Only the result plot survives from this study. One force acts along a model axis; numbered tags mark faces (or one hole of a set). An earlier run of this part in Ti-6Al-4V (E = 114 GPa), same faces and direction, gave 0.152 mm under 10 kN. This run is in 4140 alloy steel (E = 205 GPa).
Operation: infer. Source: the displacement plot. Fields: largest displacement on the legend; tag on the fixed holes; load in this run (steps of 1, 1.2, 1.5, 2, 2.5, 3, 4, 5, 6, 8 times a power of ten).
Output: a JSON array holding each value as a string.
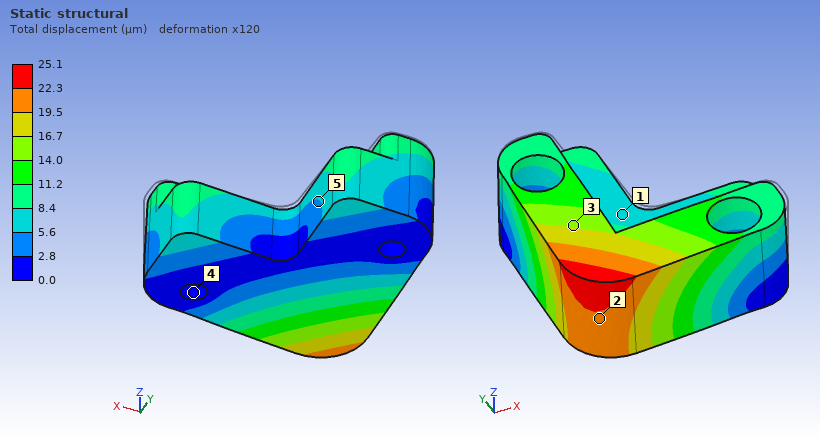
["25.1 µm", "4", "3 kN"]
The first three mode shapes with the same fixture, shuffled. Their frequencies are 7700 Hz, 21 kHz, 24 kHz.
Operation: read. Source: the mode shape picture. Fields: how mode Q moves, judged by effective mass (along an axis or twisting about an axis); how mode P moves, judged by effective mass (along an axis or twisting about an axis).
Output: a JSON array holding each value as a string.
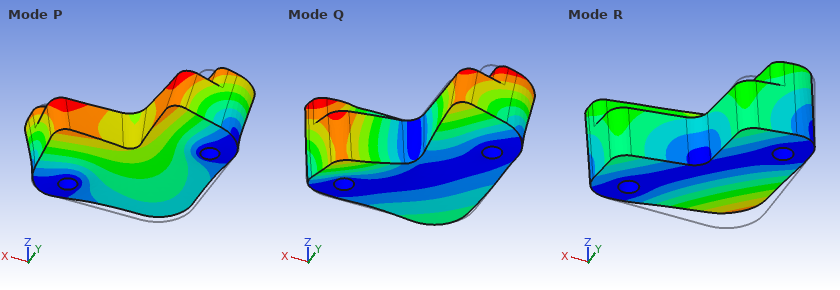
["twisting about Z", "along Z"]
